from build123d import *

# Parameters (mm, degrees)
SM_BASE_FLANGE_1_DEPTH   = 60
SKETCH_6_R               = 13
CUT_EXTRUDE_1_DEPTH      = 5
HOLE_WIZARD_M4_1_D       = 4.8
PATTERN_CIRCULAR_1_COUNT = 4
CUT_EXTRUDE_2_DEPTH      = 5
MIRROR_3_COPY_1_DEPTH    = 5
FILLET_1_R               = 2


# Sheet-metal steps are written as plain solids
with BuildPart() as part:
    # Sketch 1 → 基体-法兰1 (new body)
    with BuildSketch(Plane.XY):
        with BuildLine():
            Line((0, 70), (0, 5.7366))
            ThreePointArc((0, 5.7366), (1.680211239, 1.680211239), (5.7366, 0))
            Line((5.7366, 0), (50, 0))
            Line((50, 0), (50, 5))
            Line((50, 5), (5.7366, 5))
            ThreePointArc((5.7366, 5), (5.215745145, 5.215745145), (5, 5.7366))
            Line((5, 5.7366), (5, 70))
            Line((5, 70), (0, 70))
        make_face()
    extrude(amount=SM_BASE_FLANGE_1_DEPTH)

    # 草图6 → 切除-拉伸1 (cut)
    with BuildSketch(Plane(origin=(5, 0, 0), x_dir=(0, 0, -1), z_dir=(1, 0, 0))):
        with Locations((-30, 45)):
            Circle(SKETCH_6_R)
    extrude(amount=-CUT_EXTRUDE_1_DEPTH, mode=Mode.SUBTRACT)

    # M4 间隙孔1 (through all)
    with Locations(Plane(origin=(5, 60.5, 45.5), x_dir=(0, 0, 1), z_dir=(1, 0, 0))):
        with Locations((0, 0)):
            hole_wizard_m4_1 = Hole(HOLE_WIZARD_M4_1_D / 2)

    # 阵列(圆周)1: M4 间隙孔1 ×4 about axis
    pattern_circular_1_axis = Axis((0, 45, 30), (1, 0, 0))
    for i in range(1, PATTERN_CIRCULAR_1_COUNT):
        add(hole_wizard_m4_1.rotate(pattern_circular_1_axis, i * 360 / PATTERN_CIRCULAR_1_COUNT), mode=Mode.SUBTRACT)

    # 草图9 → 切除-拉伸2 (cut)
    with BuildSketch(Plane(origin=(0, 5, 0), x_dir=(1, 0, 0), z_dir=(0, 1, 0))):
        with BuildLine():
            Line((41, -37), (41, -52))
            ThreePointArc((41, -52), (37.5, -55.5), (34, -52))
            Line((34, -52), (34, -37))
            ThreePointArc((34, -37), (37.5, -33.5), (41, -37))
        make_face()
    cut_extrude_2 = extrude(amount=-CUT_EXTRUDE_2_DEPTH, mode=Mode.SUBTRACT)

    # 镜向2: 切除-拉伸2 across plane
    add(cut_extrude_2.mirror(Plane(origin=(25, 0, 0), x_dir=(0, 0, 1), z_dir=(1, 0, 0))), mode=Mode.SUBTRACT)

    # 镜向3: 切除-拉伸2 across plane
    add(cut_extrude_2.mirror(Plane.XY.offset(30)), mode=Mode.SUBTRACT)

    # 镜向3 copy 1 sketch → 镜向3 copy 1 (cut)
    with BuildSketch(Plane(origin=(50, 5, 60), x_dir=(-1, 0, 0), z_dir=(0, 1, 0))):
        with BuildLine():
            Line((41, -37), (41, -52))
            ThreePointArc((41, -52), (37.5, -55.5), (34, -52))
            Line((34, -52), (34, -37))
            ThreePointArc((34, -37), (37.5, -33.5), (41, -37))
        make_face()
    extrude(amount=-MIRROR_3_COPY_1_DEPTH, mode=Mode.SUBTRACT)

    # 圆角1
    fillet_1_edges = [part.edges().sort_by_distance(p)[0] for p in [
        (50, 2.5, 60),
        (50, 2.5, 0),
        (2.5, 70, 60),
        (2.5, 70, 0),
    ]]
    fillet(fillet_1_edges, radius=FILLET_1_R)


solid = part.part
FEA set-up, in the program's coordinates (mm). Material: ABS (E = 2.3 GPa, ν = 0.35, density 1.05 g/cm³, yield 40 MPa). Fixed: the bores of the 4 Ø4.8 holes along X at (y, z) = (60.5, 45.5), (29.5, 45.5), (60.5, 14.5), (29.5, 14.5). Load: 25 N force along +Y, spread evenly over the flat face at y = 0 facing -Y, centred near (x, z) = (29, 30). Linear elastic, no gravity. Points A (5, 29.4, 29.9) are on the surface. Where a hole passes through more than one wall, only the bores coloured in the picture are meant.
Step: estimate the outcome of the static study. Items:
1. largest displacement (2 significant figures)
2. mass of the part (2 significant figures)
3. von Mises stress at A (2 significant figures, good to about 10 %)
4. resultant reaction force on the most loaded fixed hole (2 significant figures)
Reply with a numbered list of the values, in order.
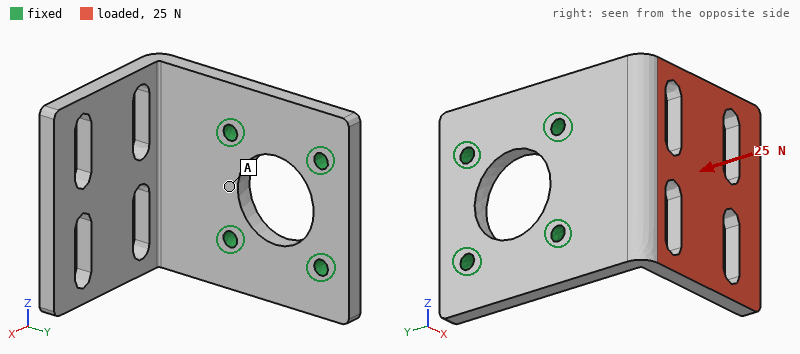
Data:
1. 1.2 mm
2. 30 g
3. 0.75 MPa
4. 12 N
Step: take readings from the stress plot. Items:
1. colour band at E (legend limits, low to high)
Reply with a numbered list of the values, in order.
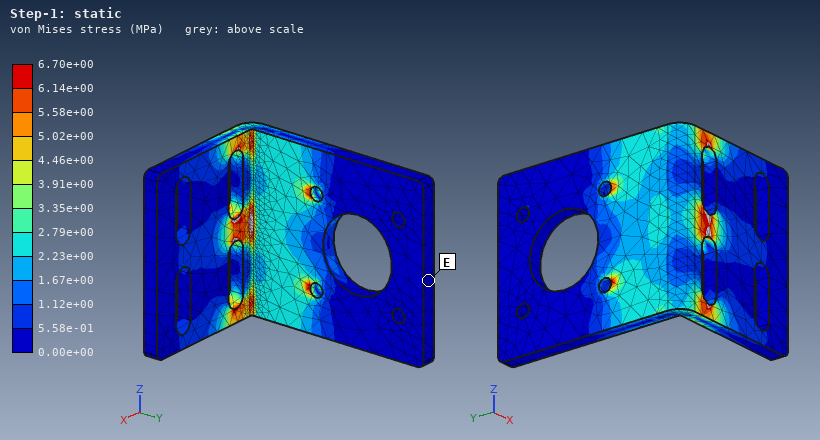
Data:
1. 0.00e+00 to 5.58e-01 MPa
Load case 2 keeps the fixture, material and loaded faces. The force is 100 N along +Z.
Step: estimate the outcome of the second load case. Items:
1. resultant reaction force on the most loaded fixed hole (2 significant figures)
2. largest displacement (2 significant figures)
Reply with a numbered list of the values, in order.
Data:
1. 110 N
2. 0.90 mm
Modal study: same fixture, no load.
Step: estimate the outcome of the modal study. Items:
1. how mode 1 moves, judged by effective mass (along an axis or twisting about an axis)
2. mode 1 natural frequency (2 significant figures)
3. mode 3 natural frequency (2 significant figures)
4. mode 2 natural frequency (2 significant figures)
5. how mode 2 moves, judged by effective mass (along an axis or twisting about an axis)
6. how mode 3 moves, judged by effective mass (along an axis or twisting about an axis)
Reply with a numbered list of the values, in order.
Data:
1. along Y
2. 260 Hz
3. 770 Hz
4. 530 Hz
5. along Z
6. along X
